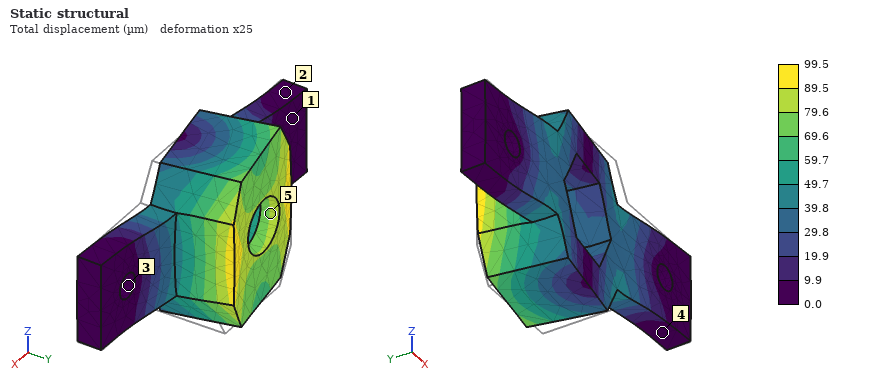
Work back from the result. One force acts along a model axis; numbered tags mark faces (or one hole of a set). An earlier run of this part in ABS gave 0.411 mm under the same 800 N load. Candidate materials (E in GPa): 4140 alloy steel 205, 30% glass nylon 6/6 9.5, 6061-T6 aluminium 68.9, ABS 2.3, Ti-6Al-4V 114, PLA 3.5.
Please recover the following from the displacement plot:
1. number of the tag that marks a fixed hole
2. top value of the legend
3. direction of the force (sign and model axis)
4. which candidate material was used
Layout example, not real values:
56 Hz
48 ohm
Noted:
3
99.5 µm
-X
30% glass nylon 6/6
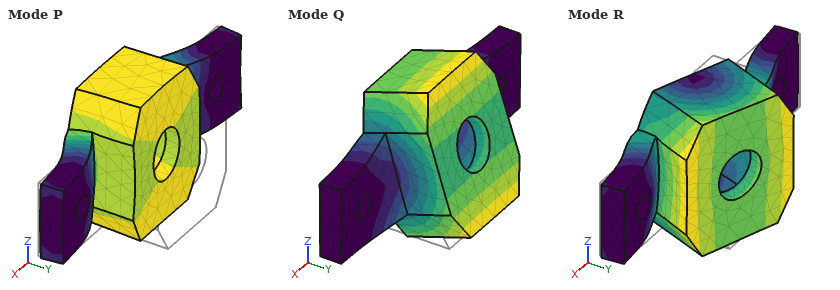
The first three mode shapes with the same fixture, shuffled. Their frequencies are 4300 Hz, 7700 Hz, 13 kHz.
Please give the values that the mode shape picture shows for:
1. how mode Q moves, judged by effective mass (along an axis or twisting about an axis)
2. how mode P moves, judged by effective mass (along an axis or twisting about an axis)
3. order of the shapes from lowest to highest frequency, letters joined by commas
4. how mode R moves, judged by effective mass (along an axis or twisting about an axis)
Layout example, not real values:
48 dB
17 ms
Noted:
along Z
along Y
Q, P, R
along X
